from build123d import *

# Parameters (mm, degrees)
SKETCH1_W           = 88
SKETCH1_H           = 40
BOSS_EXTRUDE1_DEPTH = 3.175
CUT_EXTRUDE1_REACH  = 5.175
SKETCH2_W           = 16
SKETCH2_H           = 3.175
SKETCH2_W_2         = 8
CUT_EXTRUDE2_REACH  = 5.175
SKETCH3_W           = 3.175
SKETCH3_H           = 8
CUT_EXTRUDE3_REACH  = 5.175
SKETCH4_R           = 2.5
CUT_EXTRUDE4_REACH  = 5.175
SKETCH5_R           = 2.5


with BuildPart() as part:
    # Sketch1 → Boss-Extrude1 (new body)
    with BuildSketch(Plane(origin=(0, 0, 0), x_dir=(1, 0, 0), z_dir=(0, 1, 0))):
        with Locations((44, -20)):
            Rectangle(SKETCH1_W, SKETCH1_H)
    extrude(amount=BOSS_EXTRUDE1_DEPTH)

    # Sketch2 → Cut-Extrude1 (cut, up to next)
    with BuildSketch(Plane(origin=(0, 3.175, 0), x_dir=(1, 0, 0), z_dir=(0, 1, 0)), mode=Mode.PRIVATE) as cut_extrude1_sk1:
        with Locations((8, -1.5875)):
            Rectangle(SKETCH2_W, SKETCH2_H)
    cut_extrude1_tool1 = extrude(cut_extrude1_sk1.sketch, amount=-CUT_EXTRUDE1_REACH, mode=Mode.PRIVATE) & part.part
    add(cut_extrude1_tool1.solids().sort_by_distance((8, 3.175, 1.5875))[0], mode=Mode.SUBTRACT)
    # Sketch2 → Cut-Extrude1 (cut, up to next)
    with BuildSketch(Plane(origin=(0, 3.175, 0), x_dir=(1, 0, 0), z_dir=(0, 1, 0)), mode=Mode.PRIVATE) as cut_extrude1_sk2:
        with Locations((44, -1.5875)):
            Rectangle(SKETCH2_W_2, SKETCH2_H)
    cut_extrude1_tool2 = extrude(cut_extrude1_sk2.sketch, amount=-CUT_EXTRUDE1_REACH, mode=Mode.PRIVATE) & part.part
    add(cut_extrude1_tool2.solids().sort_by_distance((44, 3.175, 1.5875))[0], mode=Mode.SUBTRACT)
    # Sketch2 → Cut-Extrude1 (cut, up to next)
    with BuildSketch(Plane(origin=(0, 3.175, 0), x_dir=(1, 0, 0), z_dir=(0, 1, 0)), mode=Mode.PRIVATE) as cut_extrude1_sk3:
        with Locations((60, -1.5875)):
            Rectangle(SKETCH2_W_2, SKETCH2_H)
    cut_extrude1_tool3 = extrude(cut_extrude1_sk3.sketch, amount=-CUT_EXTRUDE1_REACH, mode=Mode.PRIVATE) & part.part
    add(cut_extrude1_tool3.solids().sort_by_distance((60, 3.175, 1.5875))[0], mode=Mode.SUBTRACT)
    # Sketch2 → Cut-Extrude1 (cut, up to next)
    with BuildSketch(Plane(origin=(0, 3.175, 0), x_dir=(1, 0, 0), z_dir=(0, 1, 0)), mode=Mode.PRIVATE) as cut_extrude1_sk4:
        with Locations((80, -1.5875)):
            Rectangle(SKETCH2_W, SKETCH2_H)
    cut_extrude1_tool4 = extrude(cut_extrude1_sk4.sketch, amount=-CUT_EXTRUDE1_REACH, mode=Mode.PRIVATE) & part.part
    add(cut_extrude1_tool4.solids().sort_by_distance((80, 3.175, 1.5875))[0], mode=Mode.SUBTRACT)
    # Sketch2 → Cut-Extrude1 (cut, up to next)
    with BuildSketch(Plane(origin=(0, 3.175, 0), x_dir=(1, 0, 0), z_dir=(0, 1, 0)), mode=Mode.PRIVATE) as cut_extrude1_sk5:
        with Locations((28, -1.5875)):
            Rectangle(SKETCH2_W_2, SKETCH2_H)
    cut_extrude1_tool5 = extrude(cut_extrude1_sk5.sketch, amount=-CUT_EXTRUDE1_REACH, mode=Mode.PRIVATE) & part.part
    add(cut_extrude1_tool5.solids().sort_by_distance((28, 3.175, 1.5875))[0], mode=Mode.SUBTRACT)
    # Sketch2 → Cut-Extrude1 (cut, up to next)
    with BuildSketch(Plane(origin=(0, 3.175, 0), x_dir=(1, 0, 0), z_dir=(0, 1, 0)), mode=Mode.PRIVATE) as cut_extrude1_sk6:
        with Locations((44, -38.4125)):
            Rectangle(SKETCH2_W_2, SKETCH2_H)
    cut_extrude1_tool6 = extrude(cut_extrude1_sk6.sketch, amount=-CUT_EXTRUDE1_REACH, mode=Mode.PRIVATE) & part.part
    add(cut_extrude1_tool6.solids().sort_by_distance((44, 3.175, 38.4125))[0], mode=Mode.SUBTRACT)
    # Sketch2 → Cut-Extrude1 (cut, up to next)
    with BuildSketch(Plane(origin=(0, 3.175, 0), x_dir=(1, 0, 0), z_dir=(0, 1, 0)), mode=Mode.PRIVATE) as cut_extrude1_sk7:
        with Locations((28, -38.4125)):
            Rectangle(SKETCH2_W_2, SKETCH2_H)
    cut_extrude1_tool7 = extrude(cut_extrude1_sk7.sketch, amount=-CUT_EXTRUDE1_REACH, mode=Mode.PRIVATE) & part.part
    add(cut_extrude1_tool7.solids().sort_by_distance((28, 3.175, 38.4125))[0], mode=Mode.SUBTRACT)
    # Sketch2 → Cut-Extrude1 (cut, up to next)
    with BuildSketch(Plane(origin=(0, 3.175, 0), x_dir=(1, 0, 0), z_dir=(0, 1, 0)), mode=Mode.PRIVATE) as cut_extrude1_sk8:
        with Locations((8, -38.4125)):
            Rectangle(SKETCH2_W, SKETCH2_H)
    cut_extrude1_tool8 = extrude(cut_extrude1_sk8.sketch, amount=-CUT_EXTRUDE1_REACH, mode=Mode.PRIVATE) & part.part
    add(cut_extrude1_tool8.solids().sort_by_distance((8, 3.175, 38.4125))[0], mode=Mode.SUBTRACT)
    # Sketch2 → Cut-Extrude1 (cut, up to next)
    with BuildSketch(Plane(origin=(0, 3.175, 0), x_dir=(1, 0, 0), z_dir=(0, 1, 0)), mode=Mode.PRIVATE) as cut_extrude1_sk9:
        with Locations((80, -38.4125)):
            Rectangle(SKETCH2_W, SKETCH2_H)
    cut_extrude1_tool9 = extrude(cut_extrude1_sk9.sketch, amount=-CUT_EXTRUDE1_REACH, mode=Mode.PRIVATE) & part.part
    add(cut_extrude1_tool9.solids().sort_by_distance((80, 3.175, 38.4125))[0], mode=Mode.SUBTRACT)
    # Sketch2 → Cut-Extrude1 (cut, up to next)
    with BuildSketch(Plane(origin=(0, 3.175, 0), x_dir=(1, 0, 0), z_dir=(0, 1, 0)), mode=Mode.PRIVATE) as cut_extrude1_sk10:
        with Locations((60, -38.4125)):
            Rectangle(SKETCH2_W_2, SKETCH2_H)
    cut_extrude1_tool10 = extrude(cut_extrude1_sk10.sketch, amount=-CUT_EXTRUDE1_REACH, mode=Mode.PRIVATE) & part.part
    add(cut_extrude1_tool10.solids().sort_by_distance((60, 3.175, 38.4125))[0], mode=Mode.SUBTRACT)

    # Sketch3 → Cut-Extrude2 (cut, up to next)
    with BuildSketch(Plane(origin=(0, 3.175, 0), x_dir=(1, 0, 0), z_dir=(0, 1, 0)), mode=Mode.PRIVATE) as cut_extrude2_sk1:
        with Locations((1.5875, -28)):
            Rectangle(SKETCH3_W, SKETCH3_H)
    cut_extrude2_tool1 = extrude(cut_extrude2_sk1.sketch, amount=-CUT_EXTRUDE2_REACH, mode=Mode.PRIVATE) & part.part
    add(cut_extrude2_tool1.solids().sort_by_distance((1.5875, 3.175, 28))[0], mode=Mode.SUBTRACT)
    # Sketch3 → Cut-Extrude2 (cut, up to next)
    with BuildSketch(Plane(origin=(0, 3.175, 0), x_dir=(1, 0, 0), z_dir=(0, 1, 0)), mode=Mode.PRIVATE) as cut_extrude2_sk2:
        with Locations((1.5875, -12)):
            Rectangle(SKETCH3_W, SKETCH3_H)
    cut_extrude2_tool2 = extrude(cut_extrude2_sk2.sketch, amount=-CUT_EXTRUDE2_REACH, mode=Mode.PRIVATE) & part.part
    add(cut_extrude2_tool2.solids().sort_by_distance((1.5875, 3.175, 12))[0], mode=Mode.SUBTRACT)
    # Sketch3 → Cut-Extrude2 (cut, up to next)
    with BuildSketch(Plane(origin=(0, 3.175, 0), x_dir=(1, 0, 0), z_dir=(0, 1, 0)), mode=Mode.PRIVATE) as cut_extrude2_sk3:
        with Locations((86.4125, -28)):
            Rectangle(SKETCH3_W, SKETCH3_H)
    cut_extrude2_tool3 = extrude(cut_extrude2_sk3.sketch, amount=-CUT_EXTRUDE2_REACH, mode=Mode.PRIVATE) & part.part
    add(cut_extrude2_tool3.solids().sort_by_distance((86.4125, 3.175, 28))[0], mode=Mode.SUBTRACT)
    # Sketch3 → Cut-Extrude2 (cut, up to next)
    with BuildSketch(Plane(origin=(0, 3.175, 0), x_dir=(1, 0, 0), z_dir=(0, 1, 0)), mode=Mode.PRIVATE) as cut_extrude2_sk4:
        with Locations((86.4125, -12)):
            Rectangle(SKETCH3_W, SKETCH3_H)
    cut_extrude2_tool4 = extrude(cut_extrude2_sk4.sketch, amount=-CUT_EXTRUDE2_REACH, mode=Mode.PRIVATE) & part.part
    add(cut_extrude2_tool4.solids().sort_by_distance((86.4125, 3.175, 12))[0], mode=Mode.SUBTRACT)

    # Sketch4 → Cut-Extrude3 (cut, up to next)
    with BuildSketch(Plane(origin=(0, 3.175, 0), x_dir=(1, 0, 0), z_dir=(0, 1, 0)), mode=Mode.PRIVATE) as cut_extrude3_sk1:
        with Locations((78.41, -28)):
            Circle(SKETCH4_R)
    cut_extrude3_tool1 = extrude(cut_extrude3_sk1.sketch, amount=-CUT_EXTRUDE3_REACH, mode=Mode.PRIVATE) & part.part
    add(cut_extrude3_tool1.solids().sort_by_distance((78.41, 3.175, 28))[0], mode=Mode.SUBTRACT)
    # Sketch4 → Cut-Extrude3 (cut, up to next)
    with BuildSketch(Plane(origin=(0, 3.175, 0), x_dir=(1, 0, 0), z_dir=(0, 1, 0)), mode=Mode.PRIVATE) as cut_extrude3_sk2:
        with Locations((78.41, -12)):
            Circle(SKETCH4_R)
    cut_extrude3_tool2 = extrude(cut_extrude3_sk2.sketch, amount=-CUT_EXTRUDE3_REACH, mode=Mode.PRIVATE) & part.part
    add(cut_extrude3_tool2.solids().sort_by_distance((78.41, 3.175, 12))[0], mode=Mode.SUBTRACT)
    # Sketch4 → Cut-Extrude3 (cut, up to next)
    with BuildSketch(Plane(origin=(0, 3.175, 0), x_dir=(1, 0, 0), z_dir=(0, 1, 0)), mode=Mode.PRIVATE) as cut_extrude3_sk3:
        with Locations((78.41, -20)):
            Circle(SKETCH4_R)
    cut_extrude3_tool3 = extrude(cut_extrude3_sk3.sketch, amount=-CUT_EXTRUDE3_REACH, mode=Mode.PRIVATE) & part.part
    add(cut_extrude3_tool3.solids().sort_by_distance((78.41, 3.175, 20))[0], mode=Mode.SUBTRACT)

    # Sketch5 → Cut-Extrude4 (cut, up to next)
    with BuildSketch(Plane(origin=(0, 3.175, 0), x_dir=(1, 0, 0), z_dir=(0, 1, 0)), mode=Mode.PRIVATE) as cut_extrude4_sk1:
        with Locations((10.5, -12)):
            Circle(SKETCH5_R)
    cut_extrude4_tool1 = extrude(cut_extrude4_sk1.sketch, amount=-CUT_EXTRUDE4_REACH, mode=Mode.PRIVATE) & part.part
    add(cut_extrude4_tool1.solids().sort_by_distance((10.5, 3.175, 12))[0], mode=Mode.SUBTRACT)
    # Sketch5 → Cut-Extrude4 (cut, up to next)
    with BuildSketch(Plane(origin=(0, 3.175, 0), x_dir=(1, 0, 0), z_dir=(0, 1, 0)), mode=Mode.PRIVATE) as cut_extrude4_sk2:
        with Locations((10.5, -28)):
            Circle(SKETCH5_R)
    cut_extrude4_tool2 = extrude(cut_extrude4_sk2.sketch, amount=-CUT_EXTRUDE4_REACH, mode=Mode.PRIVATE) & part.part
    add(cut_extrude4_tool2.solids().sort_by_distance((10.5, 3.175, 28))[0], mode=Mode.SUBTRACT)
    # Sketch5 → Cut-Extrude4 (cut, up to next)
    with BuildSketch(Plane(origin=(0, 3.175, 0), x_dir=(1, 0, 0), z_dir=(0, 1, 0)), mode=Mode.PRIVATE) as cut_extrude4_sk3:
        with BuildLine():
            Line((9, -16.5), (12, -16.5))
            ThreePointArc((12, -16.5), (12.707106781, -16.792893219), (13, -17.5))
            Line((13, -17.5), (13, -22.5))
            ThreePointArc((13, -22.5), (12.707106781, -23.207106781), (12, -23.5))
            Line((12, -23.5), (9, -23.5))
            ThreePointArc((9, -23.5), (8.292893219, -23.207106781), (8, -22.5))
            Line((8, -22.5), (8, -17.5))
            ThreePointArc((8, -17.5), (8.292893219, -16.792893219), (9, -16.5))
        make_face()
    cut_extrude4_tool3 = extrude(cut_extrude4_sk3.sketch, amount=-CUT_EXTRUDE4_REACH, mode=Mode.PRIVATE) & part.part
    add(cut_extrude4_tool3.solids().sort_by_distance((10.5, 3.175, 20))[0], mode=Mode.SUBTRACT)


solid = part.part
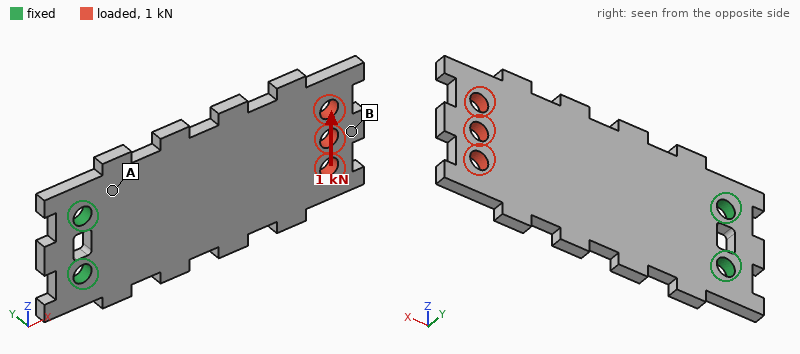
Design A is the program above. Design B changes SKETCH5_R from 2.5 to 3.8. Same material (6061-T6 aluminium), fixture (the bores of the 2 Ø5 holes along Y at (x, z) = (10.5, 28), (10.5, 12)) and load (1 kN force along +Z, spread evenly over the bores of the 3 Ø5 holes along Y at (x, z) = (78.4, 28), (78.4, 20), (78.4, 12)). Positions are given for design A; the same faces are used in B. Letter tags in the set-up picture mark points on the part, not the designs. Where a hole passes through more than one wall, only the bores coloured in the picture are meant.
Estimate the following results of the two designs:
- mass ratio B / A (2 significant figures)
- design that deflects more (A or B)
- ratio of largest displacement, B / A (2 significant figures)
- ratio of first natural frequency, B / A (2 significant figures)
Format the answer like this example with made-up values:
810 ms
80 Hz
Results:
0.98
A
0.87
1.1
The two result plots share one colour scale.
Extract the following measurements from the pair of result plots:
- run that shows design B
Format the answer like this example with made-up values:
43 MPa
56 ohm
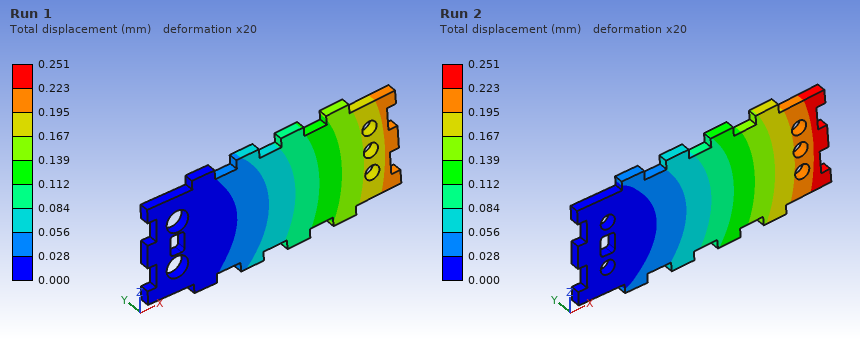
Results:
Run 1
